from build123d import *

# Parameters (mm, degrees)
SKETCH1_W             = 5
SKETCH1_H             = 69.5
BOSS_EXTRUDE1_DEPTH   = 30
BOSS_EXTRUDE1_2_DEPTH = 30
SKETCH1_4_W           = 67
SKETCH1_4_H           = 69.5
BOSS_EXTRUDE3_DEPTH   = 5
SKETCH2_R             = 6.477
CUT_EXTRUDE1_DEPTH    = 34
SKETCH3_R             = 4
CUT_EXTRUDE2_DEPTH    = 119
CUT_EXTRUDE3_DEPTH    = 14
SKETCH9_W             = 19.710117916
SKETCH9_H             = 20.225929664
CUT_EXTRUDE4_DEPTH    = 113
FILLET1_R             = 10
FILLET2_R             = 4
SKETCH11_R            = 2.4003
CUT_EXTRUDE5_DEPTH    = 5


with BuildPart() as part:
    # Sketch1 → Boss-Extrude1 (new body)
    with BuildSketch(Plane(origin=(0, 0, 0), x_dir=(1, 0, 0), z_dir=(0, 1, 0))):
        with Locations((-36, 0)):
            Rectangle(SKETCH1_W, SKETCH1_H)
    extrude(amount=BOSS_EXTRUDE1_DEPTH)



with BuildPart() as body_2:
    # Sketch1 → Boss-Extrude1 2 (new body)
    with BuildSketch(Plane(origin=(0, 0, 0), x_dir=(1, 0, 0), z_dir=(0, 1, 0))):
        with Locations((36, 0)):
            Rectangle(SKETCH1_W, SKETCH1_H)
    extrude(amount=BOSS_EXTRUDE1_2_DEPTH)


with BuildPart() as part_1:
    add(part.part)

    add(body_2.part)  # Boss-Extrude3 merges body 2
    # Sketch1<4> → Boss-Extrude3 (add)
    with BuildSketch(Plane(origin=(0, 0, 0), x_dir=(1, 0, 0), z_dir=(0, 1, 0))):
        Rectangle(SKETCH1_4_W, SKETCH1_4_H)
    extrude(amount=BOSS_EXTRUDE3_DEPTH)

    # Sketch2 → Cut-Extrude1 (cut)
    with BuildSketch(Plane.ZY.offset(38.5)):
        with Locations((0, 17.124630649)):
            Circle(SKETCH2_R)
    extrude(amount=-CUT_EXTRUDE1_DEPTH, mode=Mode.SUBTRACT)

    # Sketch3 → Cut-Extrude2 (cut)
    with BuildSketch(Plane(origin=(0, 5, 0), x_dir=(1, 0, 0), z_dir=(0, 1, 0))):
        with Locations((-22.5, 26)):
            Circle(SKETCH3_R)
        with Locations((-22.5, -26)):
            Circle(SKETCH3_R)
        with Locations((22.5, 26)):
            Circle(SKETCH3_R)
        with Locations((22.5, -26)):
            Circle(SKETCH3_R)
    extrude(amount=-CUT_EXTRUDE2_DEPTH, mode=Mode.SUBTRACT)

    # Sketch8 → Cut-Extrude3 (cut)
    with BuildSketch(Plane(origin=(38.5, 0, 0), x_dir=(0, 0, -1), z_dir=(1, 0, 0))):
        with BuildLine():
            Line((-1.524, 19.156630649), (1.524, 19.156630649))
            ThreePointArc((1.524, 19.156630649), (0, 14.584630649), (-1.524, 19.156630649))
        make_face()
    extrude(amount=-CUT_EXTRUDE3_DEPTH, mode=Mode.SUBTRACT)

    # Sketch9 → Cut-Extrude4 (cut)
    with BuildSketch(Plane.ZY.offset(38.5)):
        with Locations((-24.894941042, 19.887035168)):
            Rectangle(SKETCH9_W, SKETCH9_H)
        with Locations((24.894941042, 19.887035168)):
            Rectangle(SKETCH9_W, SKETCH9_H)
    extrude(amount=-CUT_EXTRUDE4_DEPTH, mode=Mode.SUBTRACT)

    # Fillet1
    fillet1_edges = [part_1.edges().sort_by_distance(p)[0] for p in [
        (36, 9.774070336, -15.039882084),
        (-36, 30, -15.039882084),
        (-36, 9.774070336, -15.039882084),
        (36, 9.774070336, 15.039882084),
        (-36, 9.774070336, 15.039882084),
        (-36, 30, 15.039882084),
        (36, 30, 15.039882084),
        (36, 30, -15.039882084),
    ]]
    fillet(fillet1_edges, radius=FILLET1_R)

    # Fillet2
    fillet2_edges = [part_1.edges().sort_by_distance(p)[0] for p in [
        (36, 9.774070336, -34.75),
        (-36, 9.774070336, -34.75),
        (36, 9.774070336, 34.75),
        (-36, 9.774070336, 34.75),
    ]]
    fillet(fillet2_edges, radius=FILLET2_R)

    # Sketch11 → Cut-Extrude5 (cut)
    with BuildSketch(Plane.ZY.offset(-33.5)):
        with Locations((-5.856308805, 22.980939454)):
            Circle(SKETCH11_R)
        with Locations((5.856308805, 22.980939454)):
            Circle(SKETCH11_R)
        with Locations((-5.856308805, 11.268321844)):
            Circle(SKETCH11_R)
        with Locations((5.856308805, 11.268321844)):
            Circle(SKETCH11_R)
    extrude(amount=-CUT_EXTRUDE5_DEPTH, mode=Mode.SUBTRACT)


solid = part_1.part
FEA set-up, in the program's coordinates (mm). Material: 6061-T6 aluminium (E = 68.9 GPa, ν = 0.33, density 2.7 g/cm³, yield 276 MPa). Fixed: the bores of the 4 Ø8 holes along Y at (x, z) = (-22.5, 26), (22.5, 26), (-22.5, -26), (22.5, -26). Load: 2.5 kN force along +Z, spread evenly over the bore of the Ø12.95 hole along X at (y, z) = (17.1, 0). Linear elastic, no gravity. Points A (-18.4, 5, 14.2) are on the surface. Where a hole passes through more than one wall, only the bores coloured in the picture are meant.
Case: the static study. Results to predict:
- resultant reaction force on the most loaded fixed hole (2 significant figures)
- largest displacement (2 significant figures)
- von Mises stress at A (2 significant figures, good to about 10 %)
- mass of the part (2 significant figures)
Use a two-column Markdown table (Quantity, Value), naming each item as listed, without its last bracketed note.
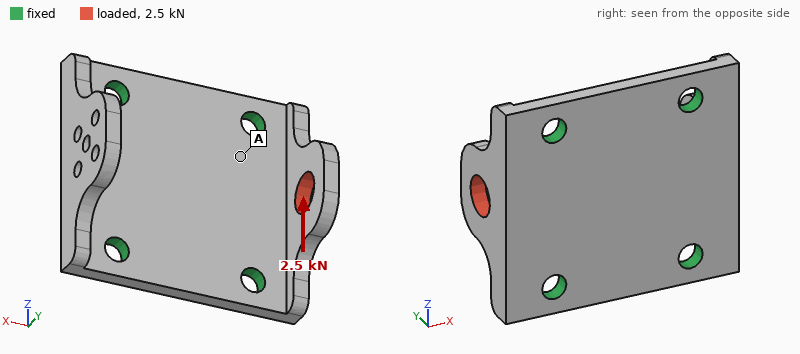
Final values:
| Quantity | Value |
|---|---|
| resultant reaction force on the most loaded fixed hole | 1.5 kN |
| largest displacement | 45 µm |
| von Mises stress at A | 8.8 MPa |
| mass of the part | 92 g |
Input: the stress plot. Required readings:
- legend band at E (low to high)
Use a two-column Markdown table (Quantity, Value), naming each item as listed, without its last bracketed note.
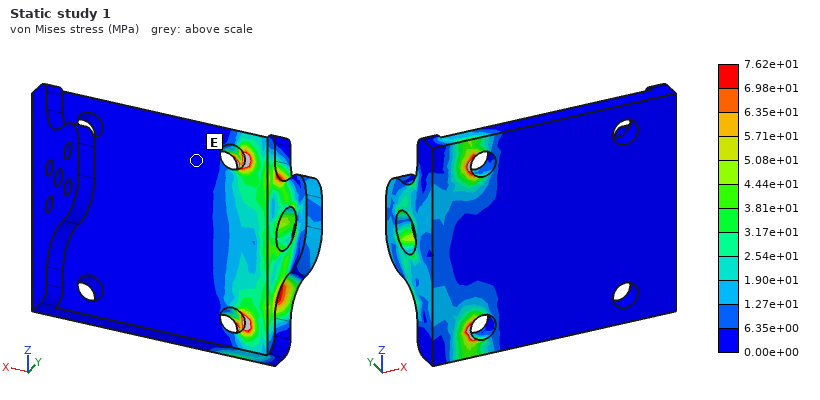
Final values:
| Quantity | Value |
|---|---|
| legend band at E | 0.00e+00 to 6.35e+00 MPa |
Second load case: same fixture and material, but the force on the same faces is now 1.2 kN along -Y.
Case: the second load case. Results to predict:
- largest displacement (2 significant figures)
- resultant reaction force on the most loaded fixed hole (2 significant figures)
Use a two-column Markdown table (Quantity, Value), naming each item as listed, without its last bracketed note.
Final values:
| Quantity | Value |
|---|---|
| largest displacement | 68 µm |
| resultant reaction force on the most loaded fixed hole | 680 N |
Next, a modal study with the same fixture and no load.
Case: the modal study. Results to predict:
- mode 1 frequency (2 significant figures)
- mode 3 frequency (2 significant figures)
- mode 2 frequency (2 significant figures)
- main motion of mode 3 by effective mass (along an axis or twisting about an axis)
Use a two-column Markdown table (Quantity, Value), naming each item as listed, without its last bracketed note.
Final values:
| Quantity | Value |
|---|---|
| mode 1 frequency | 4500 Hz |
| mode 3 frequency | 9100 Hz |
| mode 2 frequency | 4600 Hz |
| main motion of mode 3 by effective mass | along Y |
